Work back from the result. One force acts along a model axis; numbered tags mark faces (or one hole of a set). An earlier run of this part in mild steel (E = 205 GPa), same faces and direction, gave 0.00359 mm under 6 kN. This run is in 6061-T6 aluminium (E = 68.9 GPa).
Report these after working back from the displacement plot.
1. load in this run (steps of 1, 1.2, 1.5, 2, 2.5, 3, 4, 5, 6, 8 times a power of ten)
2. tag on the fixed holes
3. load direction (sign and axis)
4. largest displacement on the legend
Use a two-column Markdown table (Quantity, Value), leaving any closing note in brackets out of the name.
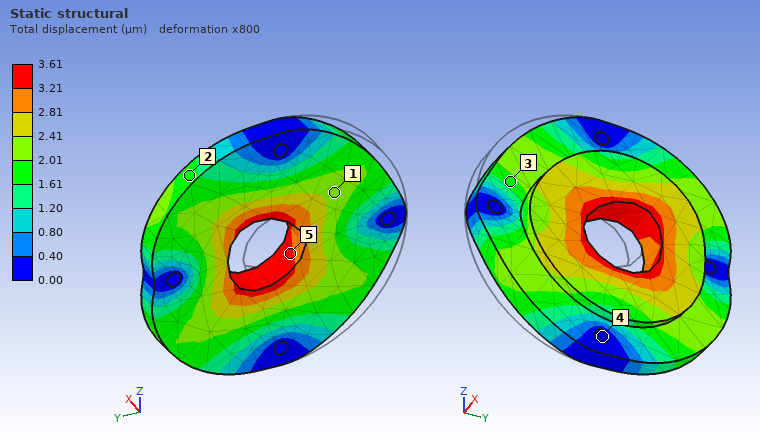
| Quantity | Value |
|---|---|
| load in this run | 2 kN |
| tag on the fixed holes | 4 |
| load direction | +Y |
| largest displacement on the legend | 3.61 µm |
